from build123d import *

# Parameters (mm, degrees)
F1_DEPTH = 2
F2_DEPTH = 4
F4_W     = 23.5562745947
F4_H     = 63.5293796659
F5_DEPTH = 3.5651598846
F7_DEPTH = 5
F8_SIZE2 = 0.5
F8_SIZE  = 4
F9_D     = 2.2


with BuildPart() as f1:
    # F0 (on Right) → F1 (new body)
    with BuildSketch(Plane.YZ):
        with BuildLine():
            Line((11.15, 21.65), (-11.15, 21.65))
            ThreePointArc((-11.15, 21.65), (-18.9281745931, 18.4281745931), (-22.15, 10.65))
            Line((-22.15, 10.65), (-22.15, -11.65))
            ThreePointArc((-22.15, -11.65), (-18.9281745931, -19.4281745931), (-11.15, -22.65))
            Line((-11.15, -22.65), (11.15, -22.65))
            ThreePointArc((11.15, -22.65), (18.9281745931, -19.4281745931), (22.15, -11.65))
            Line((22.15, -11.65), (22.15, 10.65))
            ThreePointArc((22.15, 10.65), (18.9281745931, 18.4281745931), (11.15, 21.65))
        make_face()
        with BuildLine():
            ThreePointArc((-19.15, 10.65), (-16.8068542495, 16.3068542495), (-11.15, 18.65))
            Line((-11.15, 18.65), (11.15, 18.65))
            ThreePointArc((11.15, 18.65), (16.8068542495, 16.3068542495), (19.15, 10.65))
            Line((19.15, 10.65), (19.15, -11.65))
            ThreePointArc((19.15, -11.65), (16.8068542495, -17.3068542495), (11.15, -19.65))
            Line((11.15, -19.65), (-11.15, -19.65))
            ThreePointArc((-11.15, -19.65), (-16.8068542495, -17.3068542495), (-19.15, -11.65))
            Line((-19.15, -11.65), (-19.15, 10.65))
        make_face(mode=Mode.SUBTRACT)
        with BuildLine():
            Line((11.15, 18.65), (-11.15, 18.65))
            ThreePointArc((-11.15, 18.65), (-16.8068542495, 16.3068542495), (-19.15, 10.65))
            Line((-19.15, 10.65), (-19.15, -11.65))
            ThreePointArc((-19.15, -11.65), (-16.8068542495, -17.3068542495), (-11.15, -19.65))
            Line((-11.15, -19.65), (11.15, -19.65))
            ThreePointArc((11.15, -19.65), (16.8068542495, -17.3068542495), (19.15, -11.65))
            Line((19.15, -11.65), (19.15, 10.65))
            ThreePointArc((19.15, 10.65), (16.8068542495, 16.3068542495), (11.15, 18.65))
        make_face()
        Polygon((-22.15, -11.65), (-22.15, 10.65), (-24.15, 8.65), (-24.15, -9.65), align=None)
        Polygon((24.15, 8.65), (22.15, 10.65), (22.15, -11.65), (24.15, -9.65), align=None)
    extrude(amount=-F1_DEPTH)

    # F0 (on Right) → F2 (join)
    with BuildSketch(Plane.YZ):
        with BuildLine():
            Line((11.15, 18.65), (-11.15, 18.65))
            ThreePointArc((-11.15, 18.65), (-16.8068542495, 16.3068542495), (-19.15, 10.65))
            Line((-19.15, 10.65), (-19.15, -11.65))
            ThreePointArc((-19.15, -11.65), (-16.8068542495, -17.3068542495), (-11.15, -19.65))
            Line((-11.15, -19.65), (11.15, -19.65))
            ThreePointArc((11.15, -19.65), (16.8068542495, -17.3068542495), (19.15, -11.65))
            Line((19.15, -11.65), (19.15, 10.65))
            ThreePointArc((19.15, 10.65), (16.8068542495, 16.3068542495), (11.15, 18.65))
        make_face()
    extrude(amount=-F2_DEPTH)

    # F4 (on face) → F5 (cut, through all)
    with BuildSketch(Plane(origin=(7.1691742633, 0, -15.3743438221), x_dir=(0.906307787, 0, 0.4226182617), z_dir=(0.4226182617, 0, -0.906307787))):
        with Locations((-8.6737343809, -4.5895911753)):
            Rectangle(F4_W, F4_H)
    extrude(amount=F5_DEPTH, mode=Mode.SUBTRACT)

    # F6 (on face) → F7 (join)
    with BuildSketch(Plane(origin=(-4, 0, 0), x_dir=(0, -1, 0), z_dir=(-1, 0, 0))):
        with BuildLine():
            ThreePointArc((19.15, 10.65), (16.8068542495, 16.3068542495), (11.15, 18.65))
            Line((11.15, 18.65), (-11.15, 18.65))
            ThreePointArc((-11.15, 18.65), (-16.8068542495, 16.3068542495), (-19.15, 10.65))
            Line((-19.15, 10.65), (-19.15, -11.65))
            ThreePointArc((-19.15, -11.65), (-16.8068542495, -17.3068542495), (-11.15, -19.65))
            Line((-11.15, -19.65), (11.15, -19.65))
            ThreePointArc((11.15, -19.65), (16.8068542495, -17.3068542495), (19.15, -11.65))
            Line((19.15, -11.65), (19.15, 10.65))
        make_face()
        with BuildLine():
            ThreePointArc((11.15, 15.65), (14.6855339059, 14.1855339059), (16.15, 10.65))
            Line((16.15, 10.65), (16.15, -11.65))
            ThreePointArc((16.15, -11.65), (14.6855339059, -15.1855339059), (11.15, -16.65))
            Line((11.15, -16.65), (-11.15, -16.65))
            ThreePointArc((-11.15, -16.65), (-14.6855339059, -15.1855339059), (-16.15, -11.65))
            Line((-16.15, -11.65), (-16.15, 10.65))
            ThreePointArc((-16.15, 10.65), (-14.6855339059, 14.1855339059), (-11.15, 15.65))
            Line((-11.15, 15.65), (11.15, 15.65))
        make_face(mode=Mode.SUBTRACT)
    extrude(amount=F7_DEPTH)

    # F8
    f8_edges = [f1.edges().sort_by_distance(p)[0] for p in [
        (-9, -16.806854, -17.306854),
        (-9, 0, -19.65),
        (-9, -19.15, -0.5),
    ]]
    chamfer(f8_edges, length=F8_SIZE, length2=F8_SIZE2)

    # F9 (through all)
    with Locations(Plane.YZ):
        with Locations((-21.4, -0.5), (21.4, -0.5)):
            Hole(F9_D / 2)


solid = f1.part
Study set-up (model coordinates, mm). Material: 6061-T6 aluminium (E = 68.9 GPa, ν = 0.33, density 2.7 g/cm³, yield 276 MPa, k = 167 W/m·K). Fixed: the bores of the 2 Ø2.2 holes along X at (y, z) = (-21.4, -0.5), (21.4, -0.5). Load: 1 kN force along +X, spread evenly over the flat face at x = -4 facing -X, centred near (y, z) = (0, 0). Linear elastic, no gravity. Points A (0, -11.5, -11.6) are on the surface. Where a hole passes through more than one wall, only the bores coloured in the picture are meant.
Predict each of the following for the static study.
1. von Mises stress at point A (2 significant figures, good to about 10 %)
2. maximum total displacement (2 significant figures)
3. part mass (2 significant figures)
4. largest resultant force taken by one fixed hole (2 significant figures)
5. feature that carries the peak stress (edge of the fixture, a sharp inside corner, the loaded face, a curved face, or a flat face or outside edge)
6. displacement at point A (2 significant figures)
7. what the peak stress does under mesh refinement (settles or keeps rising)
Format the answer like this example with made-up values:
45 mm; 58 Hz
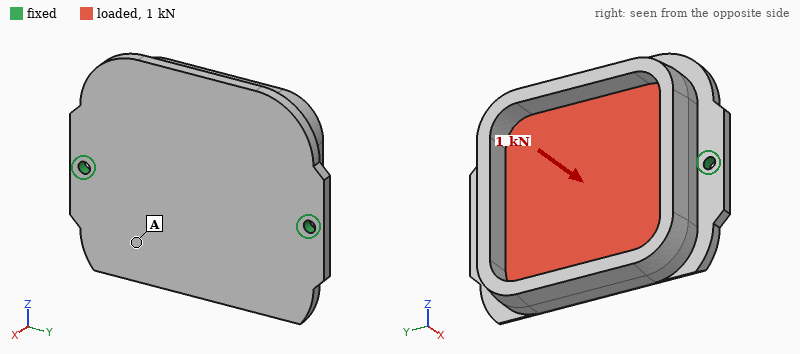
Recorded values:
16 MPa; 40 µm; 22 g; 660 N; edge of the fixture; 29 µm; keeps rising
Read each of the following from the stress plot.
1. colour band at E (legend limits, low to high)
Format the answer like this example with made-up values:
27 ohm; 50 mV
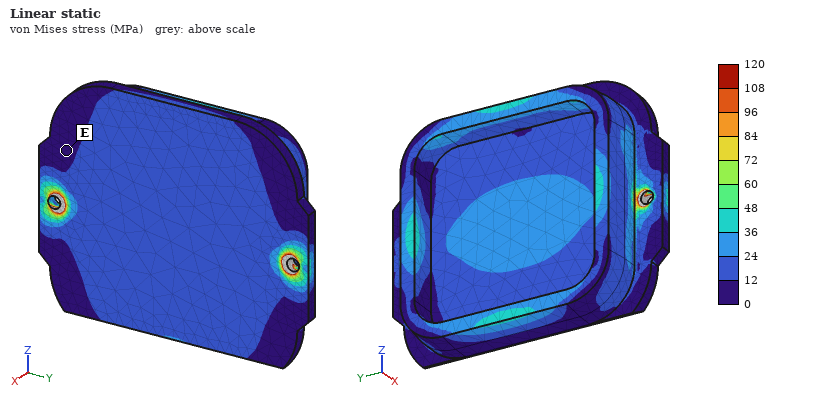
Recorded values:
0 to 12 MPa
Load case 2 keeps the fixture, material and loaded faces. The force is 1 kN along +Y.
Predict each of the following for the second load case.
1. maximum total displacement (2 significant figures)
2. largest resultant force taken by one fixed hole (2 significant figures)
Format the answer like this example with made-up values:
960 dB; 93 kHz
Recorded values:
3.7 µm; 510 N
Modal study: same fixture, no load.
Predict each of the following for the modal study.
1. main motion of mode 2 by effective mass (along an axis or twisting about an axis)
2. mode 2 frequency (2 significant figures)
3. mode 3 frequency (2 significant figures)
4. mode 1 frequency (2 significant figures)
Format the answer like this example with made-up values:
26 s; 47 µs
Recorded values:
along X; 6300 Hz; 8600 Hz; 2200 Hz
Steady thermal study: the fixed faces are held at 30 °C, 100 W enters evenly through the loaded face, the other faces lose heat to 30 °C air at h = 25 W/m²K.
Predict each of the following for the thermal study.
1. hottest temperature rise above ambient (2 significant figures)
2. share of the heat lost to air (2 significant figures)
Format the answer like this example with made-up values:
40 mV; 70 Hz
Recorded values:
72 K; 6.5 %
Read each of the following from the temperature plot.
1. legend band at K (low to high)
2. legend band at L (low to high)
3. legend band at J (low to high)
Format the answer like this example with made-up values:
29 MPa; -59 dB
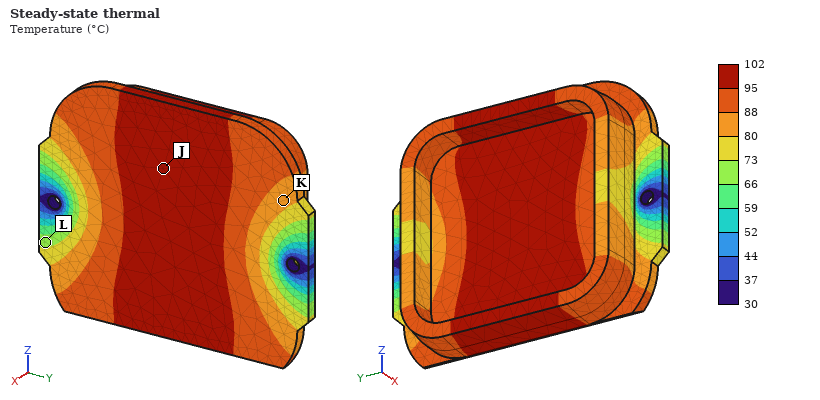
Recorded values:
80 to 88 °C; 66 to 73 °C; 95 to 102 °C
